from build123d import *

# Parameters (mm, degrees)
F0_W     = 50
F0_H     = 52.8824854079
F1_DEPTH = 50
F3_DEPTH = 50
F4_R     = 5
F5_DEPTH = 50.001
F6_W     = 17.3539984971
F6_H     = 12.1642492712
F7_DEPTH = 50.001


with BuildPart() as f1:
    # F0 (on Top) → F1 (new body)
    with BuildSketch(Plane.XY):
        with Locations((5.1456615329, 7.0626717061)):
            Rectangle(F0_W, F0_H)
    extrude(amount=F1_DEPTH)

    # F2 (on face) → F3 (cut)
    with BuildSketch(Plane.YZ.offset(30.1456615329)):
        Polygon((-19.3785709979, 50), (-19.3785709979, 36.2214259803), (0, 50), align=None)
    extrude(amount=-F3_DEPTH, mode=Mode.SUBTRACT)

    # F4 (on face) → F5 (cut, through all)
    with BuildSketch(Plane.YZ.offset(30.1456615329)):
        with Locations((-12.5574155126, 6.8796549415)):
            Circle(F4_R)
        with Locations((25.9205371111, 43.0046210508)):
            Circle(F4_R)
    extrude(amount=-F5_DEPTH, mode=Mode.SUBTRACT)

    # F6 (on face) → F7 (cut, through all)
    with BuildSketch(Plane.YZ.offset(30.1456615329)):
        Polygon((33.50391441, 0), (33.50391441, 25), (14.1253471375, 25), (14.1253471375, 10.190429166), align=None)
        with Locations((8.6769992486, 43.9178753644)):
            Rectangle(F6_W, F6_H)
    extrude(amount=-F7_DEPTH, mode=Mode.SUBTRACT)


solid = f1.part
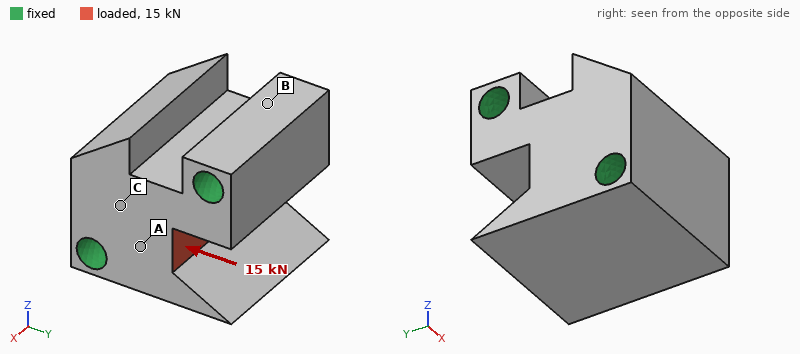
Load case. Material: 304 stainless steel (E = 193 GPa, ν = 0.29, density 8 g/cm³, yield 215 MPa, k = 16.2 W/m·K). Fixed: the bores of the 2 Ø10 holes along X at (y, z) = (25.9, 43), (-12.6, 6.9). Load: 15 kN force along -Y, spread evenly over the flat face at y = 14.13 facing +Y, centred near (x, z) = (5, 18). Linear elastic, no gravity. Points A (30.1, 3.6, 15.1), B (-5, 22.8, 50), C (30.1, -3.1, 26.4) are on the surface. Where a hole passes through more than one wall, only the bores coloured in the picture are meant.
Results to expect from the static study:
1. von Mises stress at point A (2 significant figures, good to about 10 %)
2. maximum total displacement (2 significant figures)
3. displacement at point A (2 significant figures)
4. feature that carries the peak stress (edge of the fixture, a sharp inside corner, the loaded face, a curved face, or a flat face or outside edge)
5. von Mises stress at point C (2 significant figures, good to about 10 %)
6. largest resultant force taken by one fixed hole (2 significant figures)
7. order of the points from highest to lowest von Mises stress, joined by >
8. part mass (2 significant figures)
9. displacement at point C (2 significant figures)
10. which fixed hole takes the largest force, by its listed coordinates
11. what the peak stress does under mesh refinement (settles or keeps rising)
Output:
17 MPa
4.3 µm
1.7 µm
edge of the fixture
7.0 MPa
9.9 kN
A > C > B
700 g
1.7 µm
(-12.6, 6.9)
keeps rising
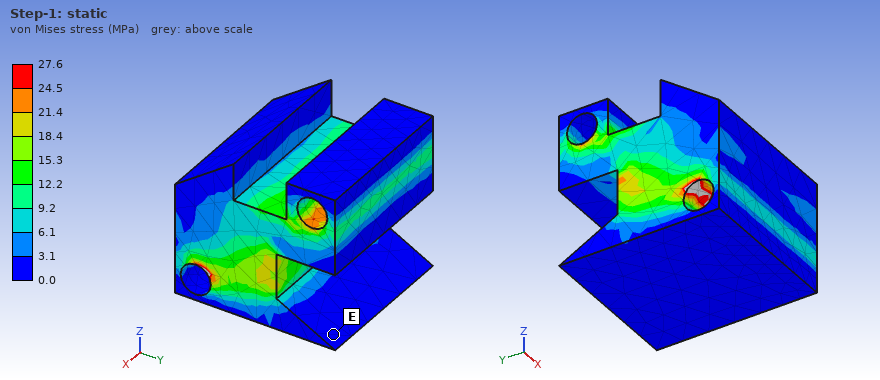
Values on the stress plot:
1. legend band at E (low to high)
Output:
0.0 to 3.1 MPa
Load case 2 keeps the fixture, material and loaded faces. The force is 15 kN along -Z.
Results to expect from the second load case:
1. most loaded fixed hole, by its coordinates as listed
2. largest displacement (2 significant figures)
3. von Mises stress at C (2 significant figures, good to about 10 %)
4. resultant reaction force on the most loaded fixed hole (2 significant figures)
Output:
(-12.6, 6.9)
8.9 µm
12 MPa
9.4 kN
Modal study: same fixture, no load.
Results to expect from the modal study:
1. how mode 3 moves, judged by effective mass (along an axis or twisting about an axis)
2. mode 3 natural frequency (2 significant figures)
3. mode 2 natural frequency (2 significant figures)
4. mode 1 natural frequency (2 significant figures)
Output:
along X
20 kHz
17 kHz
14 kHz
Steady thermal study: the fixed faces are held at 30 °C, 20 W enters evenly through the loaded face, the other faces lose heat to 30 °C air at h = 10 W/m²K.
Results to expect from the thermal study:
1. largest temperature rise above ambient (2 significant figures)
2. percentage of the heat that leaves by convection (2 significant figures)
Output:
21 K
4.1 %
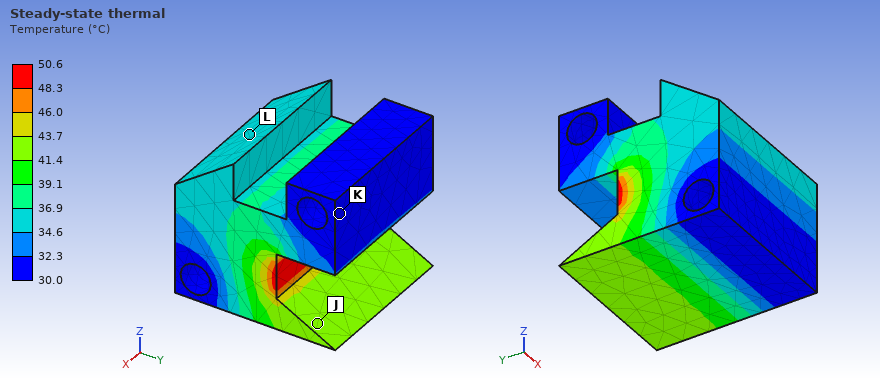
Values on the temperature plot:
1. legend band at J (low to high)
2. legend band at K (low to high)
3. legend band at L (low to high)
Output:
41.4 to 43.7 °C
30.0 to 32.3 °C
34.6 to 36.9 °C
